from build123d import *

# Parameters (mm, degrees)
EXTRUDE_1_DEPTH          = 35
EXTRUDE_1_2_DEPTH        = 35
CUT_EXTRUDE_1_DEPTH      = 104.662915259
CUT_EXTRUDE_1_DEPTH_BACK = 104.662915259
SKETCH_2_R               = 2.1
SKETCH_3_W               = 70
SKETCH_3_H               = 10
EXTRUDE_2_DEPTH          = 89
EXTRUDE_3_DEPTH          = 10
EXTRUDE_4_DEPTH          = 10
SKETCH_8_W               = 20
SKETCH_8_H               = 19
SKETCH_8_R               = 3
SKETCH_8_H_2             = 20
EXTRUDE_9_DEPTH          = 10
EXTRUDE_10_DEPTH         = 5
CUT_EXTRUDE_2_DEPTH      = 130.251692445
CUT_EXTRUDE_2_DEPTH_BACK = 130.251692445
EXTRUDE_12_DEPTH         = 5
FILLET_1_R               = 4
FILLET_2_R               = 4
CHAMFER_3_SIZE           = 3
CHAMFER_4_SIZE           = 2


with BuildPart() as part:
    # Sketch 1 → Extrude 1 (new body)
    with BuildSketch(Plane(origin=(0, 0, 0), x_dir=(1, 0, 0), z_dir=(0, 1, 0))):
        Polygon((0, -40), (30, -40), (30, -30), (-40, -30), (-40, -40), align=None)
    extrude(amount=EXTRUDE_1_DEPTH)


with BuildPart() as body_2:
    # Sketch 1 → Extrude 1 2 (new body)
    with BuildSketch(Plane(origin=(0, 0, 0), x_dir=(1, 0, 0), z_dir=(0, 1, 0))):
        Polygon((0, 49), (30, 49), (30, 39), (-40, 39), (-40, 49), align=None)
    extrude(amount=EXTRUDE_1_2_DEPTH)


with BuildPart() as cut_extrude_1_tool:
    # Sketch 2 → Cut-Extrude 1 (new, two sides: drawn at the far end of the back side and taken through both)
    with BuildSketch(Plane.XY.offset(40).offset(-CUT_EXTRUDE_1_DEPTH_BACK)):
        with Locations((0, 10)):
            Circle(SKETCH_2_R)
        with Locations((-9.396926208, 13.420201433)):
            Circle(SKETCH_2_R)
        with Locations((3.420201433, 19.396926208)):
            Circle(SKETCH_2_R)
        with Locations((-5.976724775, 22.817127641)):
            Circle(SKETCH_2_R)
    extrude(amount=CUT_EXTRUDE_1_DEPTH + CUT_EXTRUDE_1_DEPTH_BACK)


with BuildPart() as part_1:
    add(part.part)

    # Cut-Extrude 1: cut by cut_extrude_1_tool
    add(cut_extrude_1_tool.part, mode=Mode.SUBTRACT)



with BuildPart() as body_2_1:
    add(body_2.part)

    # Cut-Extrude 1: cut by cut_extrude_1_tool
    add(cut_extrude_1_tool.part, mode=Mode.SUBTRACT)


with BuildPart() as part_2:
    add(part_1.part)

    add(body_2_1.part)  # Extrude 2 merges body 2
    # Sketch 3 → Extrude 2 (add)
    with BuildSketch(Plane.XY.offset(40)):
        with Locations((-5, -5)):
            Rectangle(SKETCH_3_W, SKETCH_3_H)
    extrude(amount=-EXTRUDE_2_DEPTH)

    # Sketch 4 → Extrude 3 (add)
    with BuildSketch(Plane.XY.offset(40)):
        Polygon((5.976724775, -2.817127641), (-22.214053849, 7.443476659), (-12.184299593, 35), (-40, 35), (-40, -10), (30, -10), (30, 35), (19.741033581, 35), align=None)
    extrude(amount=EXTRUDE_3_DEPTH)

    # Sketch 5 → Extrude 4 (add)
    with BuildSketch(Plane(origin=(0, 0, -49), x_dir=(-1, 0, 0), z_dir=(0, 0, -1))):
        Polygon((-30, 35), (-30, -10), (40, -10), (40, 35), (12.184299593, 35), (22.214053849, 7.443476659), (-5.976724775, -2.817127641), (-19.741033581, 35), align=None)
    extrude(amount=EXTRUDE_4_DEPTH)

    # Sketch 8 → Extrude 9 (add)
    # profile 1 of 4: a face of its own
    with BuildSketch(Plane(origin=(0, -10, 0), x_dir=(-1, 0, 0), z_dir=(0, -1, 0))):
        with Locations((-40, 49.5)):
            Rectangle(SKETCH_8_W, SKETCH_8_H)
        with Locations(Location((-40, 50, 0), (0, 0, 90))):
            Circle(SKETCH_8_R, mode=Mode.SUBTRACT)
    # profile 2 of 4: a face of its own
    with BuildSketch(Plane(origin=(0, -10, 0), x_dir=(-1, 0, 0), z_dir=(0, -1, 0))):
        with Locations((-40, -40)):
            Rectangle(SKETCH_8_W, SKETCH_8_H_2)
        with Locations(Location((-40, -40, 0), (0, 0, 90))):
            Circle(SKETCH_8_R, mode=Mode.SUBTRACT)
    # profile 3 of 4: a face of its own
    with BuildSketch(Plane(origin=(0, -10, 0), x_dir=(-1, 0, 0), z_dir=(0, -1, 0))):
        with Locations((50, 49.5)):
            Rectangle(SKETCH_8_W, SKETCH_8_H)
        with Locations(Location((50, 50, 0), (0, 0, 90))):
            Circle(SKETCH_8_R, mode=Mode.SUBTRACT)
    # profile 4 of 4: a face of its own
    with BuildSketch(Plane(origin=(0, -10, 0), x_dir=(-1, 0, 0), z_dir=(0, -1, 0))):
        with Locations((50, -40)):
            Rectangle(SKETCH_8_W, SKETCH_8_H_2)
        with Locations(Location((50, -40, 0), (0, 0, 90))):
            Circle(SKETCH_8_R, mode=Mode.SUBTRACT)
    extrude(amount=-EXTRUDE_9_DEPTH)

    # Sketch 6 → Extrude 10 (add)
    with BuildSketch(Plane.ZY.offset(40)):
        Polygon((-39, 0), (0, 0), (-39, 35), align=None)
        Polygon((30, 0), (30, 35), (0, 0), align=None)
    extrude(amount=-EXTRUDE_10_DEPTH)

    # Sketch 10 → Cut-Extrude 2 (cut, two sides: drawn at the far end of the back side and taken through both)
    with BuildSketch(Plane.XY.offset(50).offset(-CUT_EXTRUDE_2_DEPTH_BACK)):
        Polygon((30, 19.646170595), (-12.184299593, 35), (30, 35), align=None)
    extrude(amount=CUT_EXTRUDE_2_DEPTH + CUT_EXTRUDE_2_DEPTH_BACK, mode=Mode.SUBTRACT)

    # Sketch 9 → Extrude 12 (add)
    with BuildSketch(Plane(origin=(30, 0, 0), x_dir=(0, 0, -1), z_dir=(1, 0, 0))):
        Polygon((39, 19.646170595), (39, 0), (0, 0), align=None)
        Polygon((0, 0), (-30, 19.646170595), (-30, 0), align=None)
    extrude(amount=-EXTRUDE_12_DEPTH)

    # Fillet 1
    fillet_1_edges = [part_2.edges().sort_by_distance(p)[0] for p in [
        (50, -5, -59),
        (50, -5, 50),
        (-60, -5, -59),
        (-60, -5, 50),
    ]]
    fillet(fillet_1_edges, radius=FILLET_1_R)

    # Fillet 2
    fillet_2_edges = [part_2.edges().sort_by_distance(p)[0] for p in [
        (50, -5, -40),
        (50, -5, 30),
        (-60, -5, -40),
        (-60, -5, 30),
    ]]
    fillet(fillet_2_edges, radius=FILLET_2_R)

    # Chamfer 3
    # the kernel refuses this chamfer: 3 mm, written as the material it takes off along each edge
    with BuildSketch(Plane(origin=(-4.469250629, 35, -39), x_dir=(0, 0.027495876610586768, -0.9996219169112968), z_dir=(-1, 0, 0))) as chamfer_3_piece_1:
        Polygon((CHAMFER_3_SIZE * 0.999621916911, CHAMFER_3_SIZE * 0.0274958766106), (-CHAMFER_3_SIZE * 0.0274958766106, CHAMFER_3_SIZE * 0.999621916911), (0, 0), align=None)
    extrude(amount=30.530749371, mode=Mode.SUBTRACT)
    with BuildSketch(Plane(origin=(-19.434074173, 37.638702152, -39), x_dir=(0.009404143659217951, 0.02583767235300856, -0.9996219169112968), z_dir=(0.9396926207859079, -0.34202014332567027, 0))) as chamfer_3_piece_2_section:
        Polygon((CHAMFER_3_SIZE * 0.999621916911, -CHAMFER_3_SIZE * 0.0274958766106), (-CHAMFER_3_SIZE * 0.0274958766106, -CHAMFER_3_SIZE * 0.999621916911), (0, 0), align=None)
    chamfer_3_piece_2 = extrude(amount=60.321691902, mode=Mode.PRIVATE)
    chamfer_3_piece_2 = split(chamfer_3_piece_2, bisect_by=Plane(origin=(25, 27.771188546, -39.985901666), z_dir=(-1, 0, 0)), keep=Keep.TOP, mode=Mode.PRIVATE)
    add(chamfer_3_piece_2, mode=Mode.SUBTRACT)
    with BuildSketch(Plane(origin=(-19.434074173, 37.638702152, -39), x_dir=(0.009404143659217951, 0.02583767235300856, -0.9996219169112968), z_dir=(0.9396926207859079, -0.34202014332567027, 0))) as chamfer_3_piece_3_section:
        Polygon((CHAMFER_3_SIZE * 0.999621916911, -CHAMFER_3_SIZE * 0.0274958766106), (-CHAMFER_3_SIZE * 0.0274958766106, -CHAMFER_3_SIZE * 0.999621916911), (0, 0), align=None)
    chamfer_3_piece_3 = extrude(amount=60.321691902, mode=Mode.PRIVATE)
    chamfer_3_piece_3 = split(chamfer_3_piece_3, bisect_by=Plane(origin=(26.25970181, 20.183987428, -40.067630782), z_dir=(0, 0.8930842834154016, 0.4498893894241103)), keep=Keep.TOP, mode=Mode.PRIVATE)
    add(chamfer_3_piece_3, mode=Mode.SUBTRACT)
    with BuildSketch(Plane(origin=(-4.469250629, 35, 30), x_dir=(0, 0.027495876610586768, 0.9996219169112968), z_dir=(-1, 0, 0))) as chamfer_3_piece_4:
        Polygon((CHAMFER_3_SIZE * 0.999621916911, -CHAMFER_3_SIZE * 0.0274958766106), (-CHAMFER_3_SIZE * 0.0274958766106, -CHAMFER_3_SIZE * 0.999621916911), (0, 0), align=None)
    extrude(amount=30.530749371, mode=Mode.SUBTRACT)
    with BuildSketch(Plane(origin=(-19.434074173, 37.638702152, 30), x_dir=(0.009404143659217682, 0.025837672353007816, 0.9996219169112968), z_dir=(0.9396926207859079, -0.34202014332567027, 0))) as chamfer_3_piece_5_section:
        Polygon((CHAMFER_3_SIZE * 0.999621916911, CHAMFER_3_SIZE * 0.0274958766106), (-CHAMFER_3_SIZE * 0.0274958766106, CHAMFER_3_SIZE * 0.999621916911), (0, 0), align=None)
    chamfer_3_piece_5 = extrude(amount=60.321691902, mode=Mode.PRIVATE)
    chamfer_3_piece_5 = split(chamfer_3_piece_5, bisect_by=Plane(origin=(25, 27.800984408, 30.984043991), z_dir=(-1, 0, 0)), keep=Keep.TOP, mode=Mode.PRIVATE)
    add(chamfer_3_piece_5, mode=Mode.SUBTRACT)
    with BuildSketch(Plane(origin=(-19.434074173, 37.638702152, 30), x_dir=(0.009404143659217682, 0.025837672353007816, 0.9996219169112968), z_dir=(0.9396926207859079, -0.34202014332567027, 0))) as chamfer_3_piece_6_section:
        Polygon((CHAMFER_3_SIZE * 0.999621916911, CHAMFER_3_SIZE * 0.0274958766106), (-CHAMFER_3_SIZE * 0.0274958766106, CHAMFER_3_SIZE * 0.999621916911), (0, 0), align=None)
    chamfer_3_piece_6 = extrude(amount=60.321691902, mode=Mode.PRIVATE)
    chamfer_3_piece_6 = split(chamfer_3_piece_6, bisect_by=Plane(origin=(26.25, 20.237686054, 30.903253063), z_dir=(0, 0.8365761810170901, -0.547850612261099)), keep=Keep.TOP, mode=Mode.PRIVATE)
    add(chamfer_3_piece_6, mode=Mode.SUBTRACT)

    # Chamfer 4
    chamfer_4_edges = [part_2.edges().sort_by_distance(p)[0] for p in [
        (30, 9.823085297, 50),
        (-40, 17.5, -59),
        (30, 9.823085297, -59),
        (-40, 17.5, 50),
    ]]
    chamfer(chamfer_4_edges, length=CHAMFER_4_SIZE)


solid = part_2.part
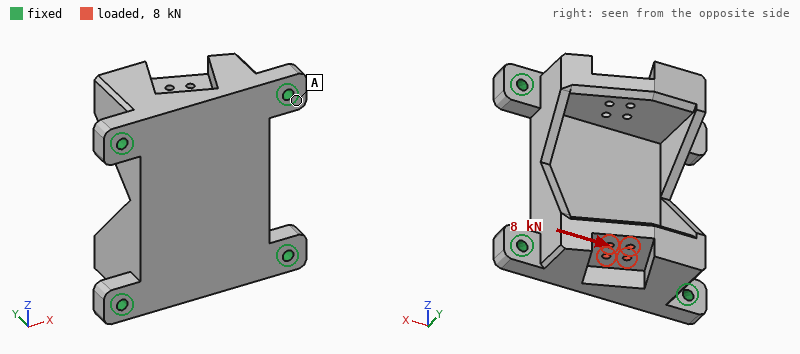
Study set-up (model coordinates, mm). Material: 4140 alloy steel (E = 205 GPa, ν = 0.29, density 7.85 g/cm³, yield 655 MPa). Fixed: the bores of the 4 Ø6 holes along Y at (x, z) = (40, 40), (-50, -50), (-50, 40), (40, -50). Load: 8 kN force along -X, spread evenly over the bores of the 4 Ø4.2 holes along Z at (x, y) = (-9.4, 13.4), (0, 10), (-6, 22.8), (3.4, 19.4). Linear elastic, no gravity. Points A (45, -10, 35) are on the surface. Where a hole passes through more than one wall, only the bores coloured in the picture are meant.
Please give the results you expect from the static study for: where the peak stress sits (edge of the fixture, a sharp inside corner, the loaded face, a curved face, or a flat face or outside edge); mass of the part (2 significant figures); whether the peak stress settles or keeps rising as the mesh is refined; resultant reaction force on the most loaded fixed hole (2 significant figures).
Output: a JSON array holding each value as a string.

["edge of the fixture", "1.3 kg", "keeps rising", "4.3 kN"]
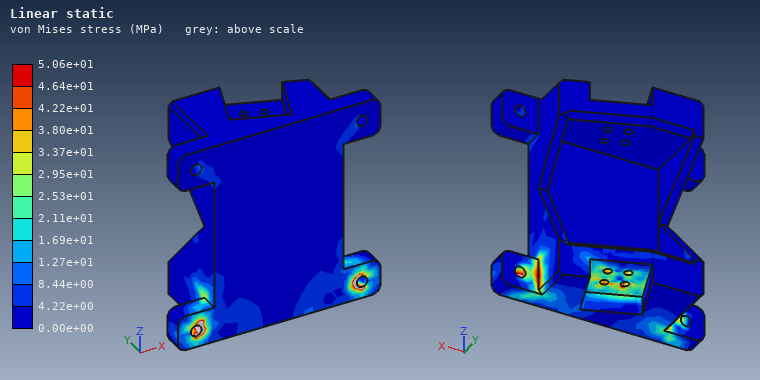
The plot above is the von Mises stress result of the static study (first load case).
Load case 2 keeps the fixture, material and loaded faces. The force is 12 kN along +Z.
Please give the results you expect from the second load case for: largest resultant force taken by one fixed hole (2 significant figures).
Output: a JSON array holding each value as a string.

["4.1 kN"]
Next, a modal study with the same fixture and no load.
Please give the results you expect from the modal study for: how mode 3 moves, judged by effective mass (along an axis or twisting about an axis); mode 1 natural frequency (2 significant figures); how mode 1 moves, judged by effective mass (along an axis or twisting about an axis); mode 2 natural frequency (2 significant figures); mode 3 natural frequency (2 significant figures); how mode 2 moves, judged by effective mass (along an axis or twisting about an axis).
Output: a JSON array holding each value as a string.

["along Y", "3200 Hz", "along Y", "5300 Hz", "6300 Hz", "along Z"]
